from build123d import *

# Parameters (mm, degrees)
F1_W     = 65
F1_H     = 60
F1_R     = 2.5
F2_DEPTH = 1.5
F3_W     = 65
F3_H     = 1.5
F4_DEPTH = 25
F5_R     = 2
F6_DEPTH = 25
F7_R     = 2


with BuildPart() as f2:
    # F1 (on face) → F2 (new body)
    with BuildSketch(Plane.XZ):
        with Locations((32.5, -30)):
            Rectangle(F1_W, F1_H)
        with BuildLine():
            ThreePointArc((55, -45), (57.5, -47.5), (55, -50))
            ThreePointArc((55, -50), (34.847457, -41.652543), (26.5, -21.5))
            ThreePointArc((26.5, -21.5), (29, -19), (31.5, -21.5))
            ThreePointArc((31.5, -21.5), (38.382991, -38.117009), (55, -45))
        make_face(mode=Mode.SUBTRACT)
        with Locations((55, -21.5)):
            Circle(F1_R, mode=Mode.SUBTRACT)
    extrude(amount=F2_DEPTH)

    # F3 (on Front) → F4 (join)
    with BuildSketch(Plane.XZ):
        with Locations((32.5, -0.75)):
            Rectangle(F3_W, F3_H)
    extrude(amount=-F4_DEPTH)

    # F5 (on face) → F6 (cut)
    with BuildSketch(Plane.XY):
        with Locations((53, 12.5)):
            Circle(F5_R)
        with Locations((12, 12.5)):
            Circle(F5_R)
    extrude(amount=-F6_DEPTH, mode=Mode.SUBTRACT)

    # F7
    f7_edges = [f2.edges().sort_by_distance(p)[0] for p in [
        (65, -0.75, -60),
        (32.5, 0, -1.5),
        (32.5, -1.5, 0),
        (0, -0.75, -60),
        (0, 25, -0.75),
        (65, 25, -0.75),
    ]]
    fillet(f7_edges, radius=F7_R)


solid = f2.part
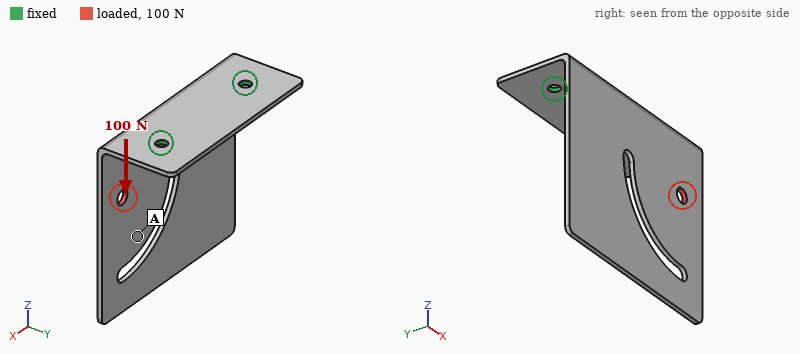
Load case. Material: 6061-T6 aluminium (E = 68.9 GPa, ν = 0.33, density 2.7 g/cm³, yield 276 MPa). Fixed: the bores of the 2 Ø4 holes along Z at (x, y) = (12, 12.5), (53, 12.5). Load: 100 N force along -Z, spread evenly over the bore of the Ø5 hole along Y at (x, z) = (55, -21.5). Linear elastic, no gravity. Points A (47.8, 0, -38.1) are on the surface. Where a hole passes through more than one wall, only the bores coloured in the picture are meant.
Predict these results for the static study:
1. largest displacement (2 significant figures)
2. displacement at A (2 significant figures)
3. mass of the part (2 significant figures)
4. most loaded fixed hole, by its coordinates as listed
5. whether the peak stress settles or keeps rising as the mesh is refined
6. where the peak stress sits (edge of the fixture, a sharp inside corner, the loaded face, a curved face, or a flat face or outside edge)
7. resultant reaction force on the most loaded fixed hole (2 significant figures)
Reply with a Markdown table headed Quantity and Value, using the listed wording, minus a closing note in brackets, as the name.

| Quantity | Value |
|---|---|
| largest displacement | 0.56 mm |
| displacement at A | 0.35 mm |
| mass of the part | 21 g |
| most loaded fixed hole, by its coordinates as listed | (53, 12.5) |
| whether the peak stress settles or keeps rising as the mesh is refined | keeps rising |
| where the peak stress sits | edge of the fixture |
| resultant reaction force on the most loaded fixed hole | 100 N |
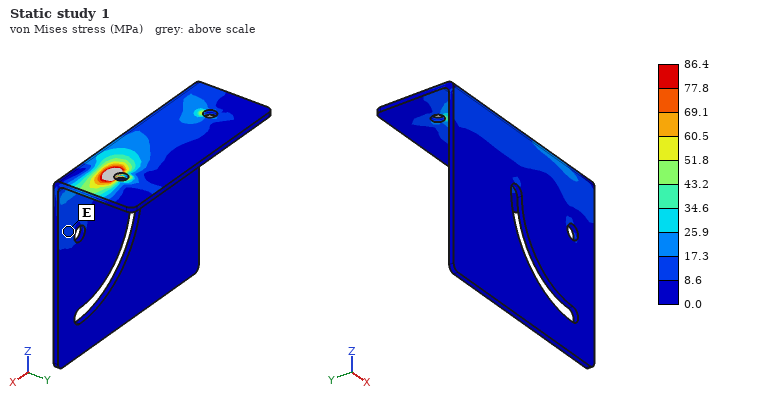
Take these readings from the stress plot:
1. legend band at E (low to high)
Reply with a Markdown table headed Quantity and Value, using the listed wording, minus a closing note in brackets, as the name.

| Quantity | Value |
|---|---|
| legend band at E | 8.6 to 17.3 MPa |
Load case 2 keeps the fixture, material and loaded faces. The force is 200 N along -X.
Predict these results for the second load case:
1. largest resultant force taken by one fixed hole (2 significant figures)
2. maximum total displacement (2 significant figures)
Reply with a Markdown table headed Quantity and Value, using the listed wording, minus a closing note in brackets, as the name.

| Quantity | Value |
|---|---|
| largest resultant force taken by one fixed hole | 150 N |
| maximum total displacement | 0.36 mm |
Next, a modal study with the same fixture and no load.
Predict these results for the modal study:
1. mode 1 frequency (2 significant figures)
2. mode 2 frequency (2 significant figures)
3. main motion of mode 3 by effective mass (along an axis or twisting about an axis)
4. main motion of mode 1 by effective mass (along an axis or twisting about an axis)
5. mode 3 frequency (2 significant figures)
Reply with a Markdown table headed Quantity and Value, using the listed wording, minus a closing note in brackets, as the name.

| Quantity | Value |
|---|---|
| mode 1 frequency | 270 Hz |
| mode 2 frequency | 640 Hz |
| main motion of mode 3 by effective mass | along X |
| main motion of mode 1 by effective mass | along Y |
| mode 3 frequency | 1200 Hz |
